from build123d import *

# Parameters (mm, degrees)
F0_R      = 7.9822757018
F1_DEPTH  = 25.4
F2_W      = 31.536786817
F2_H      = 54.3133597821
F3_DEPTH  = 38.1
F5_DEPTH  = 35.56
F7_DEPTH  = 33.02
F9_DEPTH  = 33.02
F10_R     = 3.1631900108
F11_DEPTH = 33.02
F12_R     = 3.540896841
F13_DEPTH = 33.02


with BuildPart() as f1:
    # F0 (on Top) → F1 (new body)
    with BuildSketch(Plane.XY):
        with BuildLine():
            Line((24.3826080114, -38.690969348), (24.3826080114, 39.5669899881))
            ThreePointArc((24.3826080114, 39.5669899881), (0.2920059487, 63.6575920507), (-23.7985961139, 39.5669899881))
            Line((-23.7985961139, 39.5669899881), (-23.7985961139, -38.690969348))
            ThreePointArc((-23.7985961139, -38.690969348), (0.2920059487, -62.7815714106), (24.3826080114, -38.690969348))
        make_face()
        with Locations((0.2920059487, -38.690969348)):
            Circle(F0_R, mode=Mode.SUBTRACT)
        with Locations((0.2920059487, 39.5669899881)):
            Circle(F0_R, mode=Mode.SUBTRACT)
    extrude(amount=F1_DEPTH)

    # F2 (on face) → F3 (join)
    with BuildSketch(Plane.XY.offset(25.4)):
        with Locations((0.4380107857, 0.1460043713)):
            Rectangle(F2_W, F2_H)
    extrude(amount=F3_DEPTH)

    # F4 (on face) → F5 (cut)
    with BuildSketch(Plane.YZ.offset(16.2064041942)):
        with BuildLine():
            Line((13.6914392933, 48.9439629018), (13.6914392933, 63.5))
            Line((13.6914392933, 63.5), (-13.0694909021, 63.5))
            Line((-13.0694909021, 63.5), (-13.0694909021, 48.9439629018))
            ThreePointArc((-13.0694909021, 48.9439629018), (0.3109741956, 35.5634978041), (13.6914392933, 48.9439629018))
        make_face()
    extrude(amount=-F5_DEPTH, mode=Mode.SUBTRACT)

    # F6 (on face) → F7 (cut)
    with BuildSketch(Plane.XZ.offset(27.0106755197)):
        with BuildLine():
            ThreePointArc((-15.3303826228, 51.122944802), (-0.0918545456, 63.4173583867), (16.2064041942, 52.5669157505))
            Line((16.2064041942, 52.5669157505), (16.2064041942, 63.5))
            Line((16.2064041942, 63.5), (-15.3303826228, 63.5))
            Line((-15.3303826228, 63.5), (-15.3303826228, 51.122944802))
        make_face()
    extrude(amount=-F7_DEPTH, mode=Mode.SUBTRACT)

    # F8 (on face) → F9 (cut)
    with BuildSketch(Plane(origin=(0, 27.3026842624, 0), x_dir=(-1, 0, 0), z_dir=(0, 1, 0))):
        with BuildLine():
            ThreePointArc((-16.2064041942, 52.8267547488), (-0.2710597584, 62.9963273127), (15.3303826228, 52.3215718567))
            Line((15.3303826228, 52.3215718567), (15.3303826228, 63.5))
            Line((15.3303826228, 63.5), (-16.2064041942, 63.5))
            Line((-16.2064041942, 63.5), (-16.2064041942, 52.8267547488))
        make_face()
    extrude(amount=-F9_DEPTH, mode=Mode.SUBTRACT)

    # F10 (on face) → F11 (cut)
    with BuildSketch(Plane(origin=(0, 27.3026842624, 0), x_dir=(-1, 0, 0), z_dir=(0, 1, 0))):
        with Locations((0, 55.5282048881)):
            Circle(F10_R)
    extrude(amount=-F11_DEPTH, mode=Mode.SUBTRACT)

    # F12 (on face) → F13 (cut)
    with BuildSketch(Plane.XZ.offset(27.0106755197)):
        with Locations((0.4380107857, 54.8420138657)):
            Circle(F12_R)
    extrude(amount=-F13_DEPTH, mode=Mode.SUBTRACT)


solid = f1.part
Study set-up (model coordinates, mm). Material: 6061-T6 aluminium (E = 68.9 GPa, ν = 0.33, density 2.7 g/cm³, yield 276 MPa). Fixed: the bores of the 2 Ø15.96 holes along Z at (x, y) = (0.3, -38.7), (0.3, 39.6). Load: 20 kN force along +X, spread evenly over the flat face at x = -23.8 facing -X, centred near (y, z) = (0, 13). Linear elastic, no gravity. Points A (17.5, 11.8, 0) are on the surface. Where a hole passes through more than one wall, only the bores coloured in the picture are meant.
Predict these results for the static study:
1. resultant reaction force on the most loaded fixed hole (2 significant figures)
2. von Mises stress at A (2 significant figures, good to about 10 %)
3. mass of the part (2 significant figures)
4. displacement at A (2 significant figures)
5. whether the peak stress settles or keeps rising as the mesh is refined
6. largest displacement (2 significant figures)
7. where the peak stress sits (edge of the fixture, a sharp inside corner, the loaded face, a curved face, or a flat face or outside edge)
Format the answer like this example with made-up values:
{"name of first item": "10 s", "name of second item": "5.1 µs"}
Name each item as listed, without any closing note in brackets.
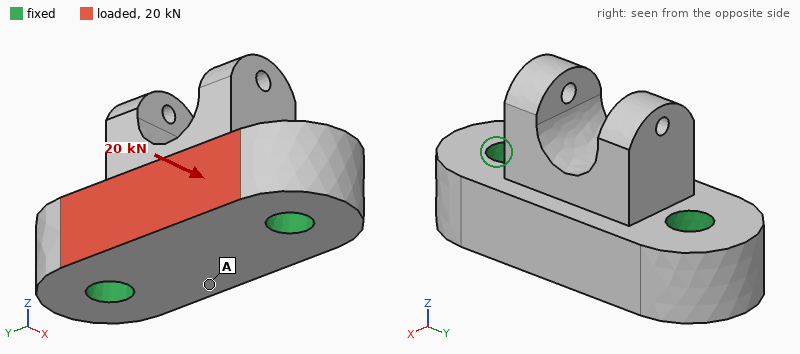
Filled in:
{"resultant reaction force on the most loaded fixed hole": "10 kN", "von Mises stress at A": "6.3 MPa", "mass of the part": "460 g", "displacement at A": "6.3 µm", "whether the peak stress settles or keeps rising as the mesh is refined": "keeps rising", "largest displacement": "11 µm", "where the peak stress sits": "edge of the fixture"}
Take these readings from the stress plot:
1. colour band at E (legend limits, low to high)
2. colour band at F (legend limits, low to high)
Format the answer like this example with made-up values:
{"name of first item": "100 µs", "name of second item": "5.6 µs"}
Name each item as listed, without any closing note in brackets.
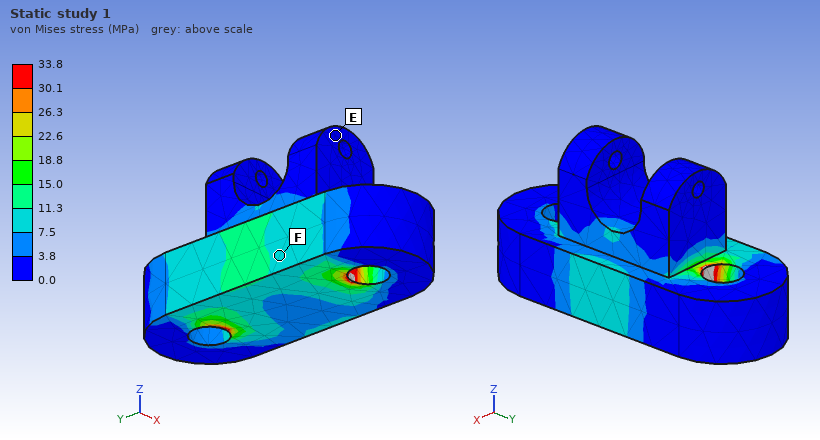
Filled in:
{"colour band at E": "0.0 to 3.8 MPa", "colour band at F": "7.5 to 11.3 MPa"}
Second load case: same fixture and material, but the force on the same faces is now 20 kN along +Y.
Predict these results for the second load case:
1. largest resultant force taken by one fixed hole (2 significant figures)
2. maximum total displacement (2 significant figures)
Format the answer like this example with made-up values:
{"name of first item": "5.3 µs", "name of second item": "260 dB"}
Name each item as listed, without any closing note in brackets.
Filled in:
{"largest resultant force taken by one fixed hole": "11 kN", "maximum total displacement": "8.4 µm"}
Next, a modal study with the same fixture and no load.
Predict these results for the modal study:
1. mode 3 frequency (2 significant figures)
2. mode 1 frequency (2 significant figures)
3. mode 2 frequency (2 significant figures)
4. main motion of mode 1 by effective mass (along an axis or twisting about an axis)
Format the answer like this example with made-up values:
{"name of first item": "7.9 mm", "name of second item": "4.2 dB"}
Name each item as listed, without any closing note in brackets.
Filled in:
{"mode 3 frequency": "12 kHz", "mode 1 frequency": "8500 Hz", "mode 2 frequency": "12 kHz", "main motion of mode 1 by effective mass": "along X"}
